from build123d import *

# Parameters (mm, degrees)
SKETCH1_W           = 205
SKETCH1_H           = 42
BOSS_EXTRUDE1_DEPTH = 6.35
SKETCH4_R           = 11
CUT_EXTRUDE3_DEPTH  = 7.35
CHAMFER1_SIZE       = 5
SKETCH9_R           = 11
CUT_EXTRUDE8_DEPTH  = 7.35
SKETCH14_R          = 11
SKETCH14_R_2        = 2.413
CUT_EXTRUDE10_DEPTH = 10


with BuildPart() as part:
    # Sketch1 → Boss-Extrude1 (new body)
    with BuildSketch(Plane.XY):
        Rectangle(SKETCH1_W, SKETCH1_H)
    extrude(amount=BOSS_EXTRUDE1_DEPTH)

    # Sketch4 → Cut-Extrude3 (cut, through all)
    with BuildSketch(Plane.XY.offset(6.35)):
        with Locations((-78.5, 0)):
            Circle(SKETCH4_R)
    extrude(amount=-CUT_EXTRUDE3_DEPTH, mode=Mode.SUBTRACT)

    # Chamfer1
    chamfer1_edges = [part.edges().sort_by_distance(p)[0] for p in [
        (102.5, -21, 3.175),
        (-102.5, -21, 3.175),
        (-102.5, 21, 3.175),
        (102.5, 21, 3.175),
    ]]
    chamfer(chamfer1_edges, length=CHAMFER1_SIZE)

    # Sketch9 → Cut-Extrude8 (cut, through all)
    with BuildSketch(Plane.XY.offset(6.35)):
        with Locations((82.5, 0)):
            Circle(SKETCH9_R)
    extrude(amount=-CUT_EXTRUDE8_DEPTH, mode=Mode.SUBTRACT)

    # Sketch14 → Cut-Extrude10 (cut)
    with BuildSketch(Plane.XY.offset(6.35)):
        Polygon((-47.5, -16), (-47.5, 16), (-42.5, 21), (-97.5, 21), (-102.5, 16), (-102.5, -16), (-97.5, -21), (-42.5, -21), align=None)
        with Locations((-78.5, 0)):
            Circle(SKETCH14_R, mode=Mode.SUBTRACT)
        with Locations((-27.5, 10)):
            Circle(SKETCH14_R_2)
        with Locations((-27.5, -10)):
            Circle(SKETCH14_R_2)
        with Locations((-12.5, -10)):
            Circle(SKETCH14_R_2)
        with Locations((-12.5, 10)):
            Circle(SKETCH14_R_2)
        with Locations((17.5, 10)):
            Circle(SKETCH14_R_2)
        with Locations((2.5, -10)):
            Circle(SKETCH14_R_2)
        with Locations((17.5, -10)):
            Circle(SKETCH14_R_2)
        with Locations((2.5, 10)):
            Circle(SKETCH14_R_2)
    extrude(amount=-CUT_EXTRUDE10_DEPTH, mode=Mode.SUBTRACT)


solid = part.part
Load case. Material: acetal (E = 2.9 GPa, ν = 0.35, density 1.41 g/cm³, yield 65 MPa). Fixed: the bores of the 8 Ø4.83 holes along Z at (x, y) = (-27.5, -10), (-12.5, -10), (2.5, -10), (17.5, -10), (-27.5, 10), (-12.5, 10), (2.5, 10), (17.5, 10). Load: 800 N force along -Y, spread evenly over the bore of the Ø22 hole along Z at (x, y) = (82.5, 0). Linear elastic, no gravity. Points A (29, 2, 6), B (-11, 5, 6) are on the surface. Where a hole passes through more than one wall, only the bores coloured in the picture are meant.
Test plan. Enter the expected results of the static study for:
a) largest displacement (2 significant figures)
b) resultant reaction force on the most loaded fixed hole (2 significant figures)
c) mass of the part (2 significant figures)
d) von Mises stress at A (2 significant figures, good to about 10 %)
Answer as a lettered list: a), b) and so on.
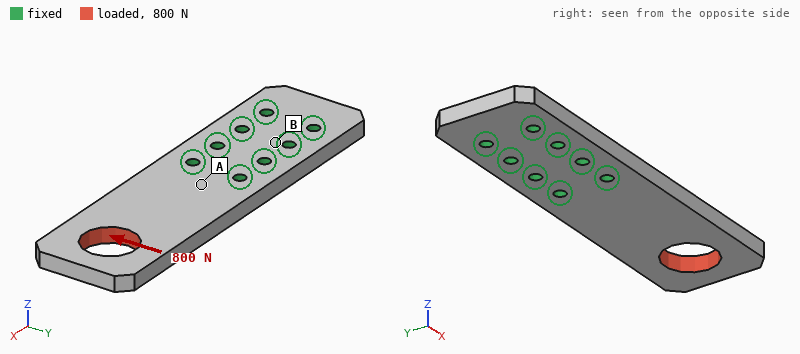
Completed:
a) 1.6 mm
b) 1.6 kN
c) 51 g
d) 11 MPa
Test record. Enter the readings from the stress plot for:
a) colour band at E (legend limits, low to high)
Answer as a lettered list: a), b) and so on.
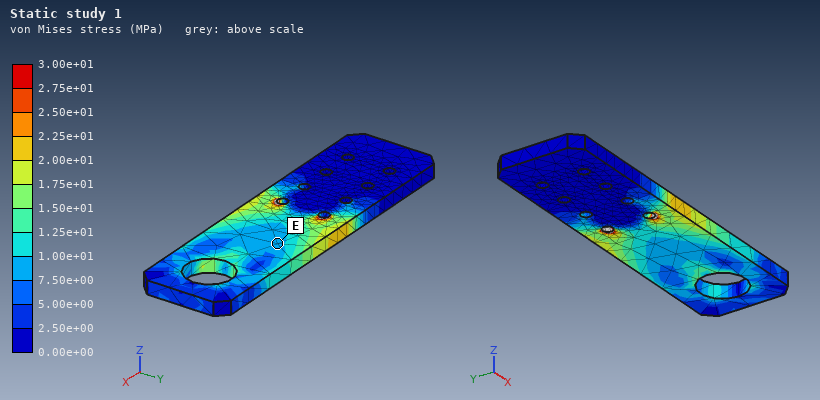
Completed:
a) 7.50e+00 to 1.00e+01 MPa
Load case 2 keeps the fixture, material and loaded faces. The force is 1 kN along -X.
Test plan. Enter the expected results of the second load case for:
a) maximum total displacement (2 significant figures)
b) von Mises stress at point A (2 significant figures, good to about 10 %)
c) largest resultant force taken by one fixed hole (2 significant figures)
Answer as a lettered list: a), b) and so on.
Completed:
a) 0.16 mm
b) 3.5 MPa
c) 410 N
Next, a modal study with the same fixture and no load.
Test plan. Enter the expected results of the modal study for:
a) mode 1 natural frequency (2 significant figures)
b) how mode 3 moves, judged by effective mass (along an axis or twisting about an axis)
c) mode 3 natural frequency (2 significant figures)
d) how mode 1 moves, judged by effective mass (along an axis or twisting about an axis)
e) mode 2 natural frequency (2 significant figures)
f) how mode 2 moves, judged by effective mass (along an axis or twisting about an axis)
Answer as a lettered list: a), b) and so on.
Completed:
a) 230 Hz
b) along Y
c) 1100 Hz
d) along Z
e) 820 Hz
f) twisting about X
